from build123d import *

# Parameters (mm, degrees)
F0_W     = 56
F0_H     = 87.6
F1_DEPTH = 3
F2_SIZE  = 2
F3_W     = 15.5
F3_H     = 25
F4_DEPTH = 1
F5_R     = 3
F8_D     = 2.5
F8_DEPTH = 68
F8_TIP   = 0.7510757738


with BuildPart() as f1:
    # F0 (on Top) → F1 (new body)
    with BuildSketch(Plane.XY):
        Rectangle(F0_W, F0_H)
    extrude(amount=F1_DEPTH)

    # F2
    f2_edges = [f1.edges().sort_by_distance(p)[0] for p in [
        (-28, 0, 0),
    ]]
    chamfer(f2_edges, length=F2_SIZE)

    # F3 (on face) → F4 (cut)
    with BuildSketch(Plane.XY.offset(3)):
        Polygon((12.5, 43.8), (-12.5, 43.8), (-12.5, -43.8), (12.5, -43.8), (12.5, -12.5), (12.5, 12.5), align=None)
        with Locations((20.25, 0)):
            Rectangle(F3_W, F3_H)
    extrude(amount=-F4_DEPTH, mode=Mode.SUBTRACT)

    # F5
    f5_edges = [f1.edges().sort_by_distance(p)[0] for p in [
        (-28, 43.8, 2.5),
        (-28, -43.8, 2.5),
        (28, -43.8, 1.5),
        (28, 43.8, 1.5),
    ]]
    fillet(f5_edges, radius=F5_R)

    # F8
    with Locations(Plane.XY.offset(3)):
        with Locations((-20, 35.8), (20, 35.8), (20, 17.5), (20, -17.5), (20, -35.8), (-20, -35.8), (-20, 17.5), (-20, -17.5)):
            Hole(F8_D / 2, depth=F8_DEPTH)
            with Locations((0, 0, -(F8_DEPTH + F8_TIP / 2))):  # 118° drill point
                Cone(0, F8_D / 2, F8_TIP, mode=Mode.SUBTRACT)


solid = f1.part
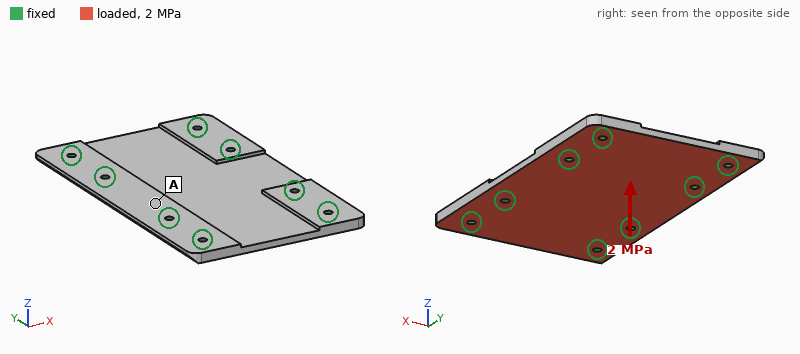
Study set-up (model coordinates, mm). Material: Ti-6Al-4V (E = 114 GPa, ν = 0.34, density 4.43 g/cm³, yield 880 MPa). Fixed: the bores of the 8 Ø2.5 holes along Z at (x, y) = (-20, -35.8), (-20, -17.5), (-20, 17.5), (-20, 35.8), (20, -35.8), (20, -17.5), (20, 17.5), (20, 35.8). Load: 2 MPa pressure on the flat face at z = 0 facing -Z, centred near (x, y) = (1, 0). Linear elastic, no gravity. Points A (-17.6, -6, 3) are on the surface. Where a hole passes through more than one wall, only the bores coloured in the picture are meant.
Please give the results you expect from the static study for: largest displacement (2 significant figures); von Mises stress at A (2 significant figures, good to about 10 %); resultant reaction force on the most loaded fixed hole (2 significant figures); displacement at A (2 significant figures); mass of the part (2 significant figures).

0.18 mm
92 MPa
1.8 kN
0.054 mm
52 g
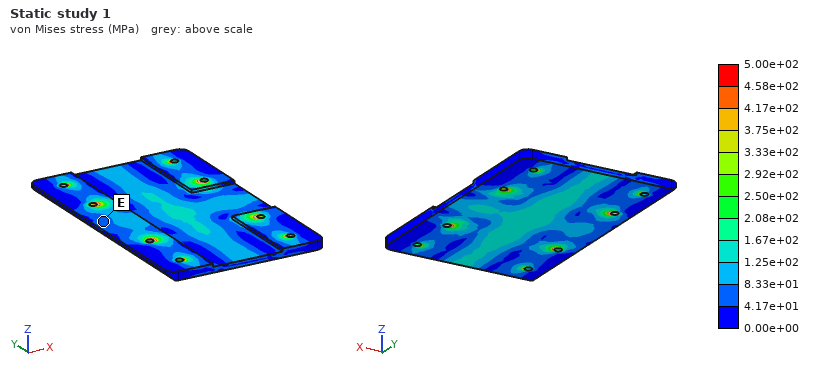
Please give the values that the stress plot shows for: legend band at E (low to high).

4.17e+01 to 8.33e+01 MPa
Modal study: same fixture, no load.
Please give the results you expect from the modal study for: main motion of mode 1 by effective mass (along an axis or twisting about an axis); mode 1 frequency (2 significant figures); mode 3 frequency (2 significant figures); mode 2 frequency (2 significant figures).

along Z
7000 Hz
9300 Hz
9100 Hz
